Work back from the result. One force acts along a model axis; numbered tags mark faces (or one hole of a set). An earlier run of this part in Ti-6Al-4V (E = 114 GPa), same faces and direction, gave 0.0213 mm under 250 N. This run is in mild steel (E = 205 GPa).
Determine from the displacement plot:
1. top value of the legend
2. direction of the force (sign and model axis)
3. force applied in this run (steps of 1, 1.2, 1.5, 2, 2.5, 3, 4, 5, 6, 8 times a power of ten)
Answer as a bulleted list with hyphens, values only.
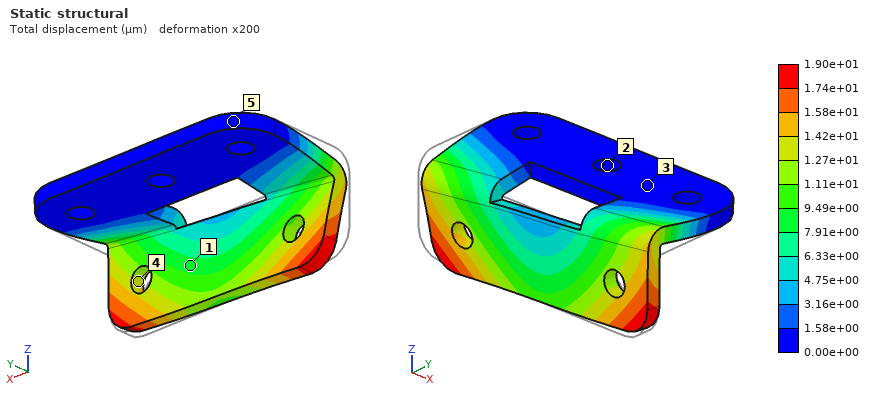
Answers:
- 1.90e+01 µm
- +X
- 400 N
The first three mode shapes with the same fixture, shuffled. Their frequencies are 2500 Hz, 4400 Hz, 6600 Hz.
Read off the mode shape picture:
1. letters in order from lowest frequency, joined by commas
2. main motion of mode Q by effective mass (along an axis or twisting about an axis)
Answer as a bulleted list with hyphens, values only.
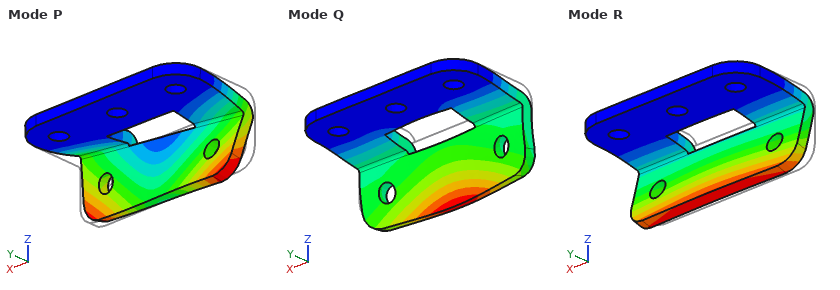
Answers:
- R, P, Q
- along Z
